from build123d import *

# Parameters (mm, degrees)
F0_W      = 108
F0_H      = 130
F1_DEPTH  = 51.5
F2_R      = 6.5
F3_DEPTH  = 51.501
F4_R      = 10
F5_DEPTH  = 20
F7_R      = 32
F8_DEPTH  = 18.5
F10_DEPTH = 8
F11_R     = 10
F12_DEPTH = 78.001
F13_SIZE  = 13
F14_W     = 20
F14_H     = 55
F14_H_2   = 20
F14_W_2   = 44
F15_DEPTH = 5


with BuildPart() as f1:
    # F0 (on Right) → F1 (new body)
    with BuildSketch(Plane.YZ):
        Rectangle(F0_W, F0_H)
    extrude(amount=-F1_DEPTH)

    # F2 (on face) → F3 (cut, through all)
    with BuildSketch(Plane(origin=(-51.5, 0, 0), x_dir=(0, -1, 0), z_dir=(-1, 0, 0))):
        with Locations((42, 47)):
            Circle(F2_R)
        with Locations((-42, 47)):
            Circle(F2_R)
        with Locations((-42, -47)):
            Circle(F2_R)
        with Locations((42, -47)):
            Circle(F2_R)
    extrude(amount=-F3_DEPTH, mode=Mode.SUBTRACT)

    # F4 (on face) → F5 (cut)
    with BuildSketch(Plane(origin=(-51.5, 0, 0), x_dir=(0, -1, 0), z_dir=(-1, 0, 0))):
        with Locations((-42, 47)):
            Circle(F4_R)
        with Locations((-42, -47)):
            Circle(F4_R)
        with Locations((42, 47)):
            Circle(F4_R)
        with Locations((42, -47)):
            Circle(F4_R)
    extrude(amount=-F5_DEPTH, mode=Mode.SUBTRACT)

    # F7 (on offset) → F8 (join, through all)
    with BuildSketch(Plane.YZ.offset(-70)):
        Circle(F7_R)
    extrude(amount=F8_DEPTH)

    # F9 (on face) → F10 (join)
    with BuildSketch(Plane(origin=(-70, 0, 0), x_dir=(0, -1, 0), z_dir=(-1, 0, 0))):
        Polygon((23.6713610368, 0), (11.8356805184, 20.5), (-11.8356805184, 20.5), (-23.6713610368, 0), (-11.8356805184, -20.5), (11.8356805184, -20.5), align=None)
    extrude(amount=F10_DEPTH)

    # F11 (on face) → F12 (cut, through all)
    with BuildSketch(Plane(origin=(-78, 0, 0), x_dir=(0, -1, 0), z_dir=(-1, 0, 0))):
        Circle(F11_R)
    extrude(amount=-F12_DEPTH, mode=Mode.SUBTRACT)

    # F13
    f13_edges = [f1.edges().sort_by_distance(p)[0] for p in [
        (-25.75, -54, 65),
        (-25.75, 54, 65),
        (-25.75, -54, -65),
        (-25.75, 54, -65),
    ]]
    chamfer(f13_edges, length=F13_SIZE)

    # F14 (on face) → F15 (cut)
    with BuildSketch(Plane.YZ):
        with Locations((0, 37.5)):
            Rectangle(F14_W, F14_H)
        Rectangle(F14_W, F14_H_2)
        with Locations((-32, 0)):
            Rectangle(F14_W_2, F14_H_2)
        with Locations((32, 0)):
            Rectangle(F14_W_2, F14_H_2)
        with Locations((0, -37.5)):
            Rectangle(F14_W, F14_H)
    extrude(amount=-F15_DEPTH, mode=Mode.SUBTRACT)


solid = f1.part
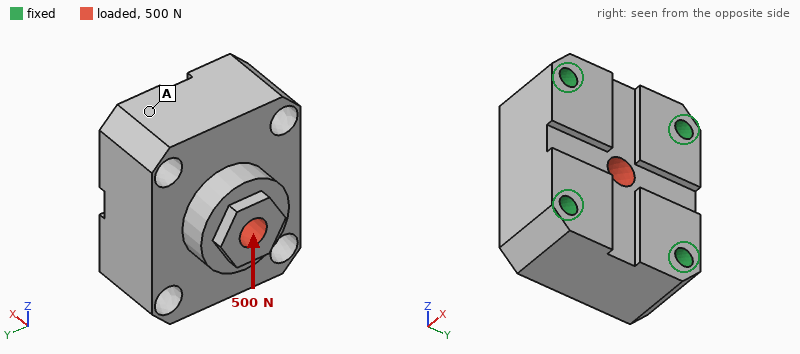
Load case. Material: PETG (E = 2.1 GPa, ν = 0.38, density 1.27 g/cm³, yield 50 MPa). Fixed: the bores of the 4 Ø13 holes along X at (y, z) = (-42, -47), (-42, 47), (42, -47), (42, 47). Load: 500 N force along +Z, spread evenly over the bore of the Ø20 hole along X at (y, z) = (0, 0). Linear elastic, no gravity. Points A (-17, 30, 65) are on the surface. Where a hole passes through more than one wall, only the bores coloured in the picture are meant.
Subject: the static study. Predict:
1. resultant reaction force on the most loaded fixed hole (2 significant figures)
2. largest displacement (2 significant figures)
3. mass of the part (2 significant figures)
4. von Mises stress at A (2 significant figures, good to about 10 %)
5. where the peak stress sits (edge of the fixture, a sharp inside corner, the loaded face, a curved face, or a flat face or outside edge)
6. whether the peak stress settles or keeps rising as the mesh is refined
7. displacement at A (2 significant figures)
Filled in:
150 N
7.8 µm
880 g
0.060 MPa
edge of the fixture
keeps rising
1.4 µm
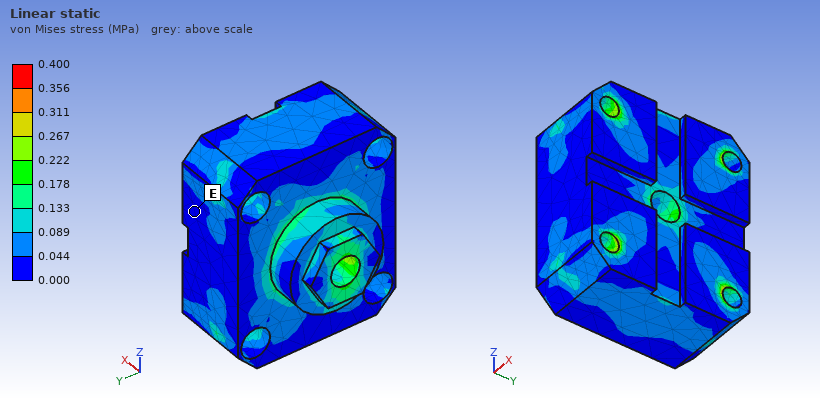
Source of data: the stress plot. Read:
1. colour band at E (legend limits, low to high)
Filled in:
0.000 to 0.044 MPa
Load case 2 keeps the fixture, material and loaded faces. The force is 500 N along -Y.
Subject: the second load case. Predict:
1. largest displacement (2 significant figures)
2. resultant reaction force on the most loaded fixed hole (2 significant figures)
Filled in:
8.9 µm
160 N
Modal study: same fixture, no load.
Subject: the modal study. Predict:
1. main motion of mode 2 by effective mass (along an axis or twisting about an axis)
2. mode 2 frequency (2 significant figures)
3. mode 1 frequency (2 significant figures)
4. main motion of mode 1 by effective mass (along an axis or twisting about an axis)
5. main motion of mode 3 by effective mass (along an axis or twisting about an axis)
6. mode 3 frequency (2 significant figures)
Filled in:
along Y
2600 Hz
2400 Hz
along X
along Z
2700 Hz
